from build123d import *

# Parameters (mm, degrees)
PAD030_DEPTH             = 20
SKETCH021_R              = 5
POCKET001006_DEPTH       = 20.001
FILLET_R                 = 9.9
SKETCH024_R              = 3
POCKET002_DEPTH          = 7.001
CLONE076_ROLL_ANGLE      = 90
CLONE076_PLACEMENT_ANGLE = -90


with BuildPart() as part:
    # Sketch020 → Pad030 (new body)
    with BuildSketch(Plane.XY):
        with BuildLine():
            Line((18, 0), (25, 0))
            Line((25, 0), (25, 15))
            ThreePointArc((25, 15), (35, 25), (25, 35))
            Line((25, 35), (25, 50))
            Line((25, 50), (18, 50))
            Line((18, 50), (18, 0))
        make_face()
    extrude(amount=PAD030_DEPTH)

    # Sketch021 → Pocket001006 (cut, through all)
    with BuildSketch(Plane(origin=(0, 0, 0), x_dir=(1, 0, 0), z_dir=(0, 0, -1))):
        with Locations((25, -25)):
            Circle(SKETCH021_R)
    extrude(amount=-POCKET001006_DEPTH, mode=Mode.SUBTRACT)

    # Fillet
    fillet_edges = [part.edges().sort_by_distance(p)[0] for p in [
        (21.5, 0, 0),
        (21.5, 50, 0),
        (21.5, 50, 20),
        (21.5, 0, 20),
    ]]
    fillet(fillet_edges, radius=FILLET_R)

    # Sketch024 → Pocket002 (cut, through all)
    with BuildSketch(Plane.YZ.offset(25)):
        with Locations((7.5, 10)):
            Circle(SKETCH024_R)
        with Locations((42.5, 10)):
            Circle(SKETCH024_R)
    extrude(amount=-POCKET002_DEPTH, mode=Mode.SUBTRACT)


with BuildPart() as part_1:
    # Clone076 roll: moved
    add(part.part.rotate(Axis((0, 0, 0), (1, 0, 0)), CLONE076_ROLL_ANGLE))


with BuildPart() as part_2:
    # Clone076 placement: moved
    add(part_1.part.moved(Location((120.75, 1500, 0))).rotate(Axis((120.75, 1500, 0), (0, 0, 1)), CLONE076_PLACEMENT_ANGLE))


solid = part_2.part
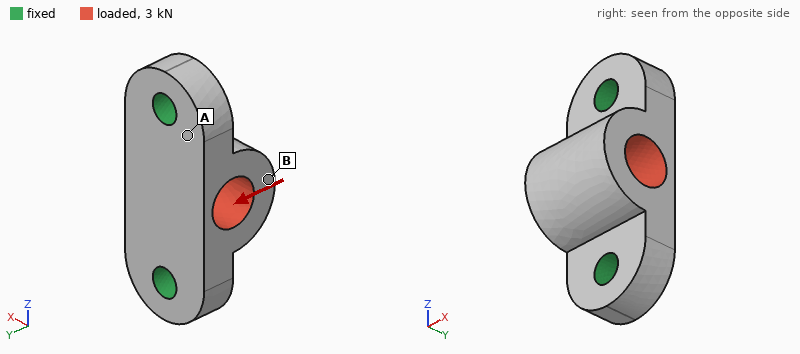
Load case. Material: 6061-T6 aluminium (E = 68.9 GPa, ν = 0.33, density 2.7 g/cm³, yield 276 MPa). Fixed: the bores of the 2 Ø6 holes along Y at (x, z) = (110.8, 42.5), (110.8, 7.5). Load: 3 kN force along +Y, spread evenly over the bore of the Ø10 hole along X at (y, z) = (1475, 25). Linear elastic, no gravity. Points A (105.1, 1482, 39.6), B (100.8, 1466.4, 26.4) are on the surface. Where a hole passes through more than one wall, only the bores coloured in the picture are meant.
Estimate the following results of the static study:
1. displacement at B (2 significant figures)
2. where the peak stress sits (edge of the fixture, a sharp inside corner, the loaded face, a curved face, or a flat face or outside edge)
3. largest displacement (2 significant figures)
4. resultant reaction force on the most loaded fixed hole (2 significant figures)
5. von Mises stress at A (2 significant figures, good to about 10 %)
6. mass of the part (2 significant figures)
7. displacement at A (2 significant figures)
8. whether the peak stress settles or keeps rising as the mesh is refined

8.9 µm
edge of the fixture
15 µm
1.5 kN
17 MPa
20 g
3.3 µm
keeps rising
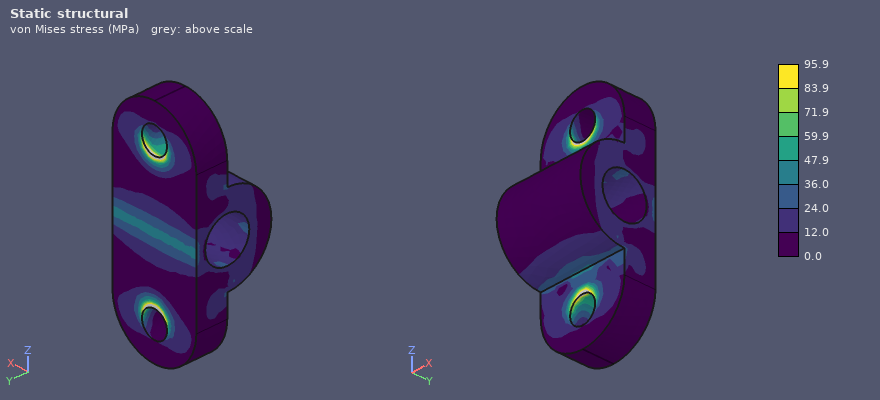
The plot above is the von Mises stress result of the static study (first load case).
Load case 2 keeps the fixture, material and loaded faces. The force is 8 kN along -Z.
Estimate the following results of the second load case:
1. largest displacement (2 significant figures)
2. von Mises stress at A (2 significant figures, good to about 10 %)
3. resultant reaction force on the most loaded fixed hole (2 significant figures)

15 µm
11 MPa
4.1 kN
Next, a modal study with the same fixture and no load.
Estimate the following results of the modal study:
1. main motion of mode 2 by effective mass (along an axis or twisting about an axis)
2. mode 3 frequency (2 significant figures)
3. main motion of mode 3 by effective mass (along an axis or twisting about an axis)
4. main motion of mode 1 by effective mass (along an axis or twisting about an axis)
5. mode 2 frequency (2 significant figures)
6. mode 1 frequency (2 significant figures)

along Y
32 kHz
along X
along X
26 kHz
17 kHz
